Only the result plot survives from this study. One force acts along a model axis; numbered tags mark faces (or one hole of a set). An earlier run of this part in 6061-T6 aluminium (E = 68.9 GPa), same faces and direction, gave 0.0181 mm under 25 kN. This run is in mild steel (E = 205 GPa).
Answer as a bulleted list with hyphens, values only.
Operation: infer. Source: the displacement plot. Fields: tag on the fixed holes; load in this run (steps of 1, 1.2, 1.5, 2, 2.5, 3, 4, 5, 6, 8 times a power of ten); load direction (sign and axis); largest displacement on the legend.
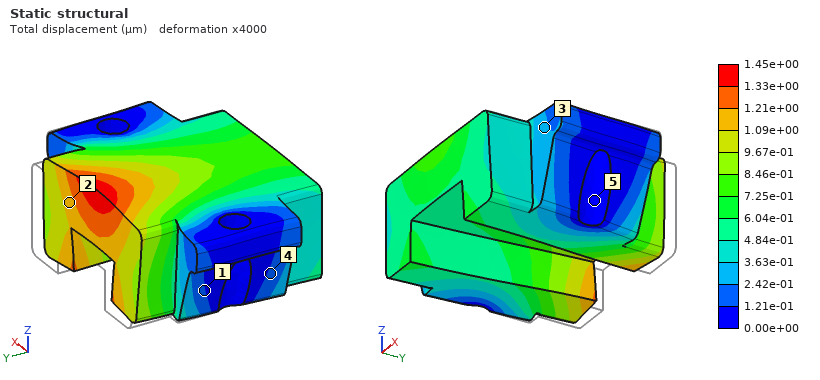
- 5
- 6 kN
- -Y
- 1.45e+00 µm
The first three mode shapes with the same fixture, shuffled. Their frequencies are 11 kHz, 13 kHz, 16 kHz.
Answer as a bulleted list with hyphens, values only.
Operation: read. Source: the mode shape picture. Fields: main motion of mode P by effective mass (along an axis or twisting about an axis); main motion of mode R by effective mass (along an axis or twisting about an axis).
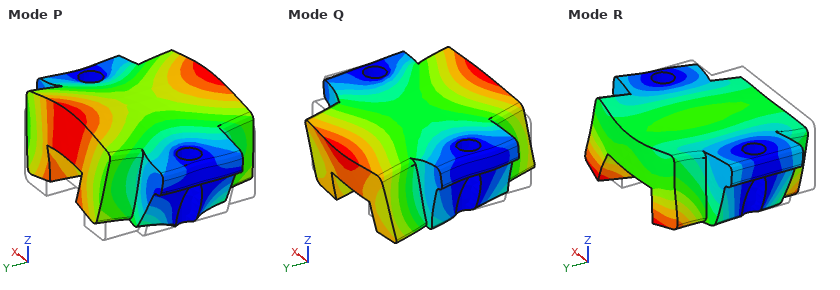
- along Z
- along Y
